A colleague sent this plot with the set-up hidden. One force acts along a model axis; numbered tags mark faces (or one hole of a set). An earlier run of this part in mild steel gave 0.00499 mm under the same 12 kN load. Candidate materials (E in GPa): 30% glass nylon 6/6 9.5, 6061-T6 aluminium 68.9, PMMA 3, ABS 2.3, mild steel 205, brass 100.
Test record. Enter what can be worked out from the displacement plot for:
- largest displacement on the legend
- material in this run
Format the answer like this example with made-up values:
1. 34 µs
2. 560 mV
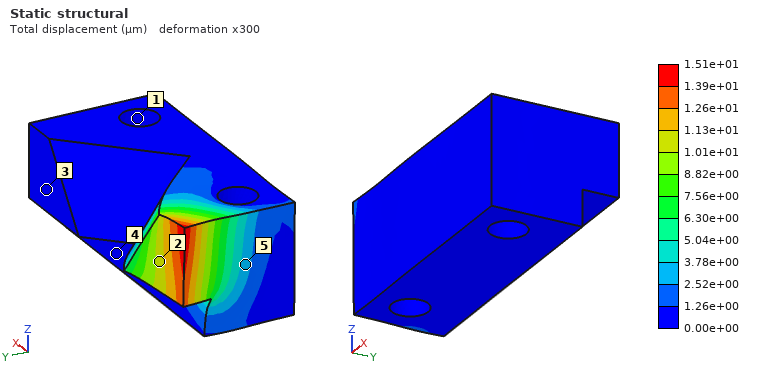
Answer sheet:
1. 1.51e+01 µm
2. 6061-T6 aluminium
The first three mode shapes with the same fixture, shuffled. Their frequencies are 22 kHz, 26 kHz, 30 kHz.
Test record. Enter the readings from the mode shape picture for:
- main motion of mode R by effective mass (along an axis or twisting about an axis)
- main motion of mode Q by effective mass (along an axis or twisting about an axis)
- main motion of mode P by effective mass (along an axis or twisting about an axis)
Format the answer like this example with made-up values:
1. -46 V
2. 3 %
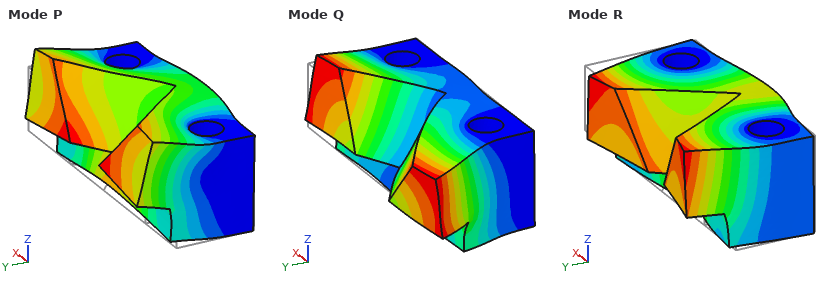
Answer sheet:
1. along Y
2. along X
3. along Z
